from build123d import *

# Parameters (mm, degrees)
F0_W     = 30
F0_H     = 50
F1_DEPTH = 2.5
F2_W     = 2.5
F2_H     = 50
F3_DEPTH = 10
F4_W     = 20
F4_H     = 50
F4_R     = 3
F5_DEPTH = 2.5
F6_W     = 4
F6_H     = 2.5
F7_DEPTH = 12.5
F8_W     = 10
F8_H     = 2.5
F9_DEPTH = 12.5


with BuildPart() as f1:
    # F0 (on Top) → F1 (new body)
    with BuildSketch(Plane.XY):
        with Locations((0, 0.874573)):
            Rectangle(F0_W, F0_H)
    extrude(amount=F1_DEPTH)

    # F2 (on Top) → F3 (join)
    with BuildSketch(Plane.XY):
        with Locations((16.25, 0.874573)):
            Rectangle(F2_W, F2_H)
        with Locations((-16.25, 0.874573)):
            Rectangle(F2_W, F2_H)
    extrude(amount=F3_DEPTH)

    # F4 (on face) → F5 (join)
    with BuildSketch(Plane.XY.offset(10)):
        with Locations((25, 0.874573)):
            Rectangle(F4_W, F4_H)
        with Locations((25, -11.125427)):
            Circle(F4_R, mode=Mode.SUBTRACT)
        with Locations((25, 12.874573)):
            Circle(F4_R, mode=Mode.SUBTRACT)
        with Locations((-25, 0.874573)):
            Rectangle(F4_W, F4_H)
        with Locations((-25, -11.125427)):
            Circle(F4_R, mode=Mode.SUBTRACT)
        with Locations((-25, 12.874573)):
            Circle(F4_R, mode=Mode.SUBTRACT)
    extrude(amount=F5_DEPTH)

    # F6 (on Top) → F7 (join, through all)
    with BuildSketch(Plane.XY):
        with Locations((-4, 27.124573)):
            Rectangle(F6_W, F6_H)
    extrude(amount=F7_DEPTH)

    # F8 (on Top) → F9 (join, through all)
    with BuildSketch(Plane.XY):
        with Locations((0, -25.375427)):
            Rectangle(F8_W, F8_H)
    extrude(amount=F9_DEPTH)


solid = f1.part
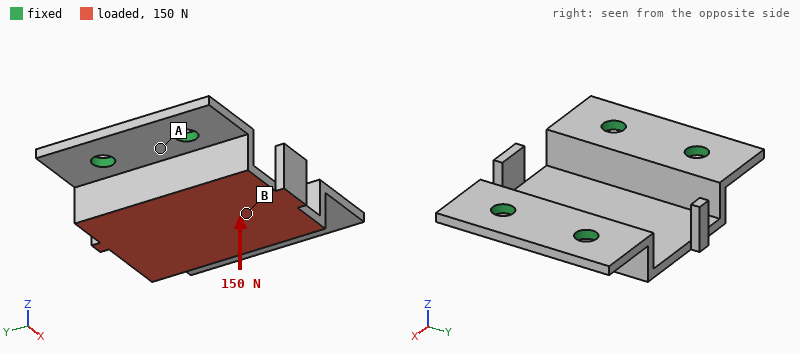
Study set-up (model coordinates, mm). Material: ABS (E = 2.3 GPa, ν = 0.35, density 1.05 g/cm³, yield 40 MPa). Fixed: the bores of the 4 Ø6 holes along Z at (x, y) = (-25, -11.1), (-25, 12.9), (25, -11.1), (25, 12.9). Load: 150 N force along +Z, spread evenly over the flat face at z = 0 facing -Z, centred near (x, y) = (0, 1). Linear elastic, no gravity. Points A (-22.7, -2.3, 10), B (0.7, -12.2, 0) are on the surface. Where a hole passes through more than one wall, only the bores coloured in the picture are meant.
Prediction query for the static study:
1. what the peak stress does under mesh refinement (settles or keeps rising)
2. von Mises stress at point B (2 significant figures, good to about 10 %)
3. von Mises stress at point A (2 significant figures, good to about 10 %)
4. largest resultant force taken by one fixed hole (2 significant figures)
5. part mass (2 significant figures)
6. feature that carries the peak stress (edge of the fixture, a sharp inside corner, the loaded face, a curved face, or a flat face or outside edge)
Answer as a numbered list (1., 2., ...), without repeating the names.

1. keeps rising
2. 3.9 MPa
3. 0.92 MPa
4. 49 N
5. 12 g
6. edge of the fixture
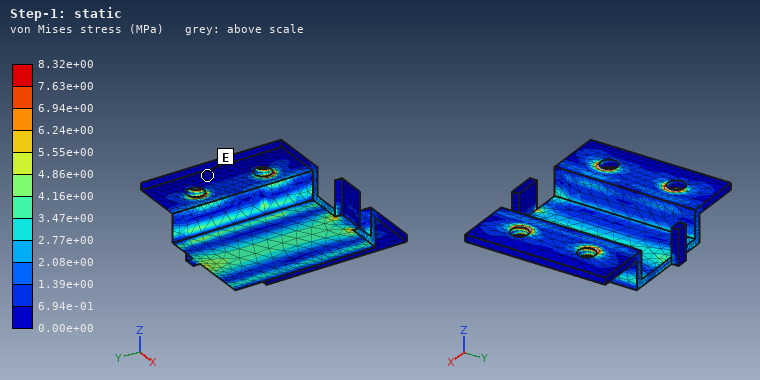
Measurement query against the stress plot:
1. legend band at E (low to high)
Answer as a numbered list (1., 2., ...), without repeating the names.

1. 0.00e+00 to 6.94e-01 MPa
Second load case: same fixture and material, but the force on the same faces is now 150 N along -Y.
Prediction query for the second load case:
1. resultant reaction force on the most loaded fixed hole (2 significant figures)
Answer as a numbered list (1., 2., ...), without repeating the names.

1. 57 N
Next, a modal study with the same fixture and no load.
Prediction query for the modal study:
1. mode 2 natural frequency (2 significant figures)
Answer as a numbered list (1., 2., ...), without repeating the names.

1. 1900 Hz
